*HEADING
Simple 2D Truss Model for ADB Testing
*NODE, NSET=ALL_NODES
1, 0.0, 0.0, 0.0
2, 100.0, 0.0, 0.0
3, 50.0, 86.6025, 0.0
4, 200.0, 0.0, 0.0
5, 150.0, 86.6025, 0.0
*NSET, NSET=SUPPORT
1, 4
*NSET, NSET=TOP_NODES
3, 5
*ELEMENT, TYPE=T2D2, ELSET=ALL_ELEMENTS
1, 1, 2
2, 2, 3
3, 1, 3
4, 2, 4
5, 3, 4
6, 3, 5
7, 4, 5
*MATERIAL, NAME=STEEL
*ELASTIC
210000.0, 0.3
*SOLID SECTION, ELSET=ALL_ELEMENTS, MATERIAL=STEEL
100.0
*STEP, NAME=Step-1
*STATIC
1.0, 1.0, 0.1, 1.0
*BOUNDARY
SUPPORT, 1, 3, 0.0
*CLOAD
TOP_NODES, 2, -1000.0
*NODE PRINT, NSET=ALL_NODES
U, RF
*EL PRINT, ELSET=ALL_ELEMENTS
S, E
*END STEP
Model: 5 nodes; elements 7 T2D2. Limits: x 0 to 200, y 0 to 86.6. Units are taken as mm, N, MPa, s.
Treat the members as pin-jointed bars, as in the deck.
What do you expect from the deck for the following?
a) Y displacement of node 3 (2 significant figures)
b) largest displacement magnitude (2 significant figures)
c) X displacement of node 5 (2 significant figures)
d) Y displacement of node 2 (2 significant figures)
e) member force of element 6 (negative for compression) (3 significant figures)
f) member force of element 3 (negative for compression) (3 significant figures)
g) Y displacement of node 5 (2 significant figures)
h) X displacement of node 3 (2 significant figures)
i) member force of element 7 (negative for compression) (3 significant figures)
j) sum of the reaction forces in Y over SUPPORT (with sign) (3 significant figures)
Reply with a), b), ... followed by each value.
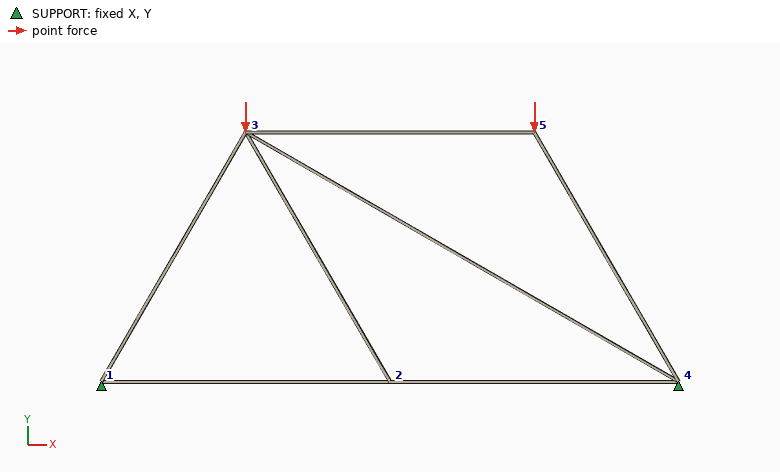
a) -0.0048 mm
b) 0.011 mm
c) -0.0055 mm
d) -0.0032 mm
e) -577 N
f) -1150 N
g) -0.0095 mm
h) -0.0027 mm
i) -1150 N
j) 2000 N
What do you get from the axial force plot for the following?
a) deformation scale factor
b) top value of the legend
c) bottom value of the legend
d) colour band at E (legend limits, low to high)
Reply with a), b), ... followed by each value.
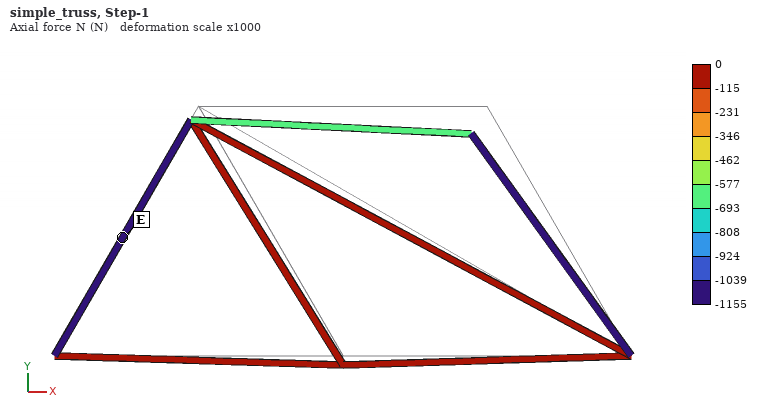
a) 1000
b) 0 N
c) -1155 N
d) -1155 to -1039 N
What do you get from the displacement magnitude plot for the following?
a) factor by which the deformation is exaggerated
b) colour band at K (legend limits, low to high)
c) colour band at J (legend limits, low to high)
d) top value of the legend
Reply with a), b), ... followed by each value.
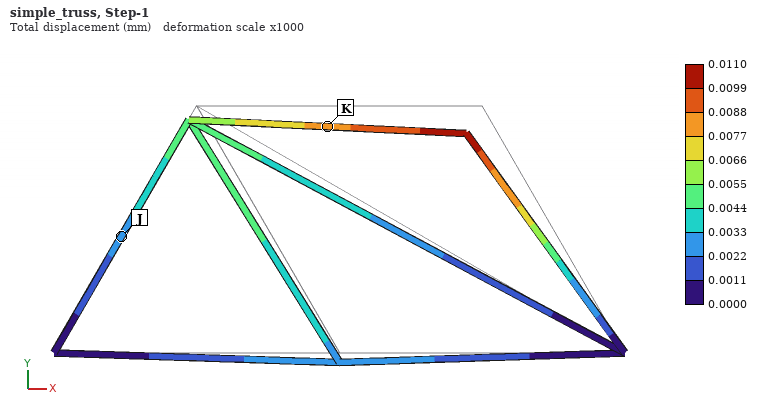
a) 1000
b) 0.0077 to 0.0088 mm
c) 0.0022 to 0.0033 mm
d) 0.0110 mm
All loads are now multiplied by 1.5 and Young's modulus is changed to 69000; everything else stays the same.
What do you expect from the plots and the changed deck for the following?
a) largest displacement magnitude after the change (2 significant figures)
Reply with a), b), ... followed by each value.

a) 0.050 mm
